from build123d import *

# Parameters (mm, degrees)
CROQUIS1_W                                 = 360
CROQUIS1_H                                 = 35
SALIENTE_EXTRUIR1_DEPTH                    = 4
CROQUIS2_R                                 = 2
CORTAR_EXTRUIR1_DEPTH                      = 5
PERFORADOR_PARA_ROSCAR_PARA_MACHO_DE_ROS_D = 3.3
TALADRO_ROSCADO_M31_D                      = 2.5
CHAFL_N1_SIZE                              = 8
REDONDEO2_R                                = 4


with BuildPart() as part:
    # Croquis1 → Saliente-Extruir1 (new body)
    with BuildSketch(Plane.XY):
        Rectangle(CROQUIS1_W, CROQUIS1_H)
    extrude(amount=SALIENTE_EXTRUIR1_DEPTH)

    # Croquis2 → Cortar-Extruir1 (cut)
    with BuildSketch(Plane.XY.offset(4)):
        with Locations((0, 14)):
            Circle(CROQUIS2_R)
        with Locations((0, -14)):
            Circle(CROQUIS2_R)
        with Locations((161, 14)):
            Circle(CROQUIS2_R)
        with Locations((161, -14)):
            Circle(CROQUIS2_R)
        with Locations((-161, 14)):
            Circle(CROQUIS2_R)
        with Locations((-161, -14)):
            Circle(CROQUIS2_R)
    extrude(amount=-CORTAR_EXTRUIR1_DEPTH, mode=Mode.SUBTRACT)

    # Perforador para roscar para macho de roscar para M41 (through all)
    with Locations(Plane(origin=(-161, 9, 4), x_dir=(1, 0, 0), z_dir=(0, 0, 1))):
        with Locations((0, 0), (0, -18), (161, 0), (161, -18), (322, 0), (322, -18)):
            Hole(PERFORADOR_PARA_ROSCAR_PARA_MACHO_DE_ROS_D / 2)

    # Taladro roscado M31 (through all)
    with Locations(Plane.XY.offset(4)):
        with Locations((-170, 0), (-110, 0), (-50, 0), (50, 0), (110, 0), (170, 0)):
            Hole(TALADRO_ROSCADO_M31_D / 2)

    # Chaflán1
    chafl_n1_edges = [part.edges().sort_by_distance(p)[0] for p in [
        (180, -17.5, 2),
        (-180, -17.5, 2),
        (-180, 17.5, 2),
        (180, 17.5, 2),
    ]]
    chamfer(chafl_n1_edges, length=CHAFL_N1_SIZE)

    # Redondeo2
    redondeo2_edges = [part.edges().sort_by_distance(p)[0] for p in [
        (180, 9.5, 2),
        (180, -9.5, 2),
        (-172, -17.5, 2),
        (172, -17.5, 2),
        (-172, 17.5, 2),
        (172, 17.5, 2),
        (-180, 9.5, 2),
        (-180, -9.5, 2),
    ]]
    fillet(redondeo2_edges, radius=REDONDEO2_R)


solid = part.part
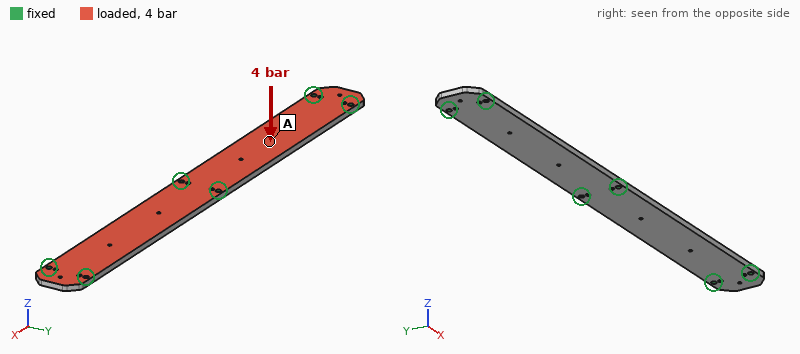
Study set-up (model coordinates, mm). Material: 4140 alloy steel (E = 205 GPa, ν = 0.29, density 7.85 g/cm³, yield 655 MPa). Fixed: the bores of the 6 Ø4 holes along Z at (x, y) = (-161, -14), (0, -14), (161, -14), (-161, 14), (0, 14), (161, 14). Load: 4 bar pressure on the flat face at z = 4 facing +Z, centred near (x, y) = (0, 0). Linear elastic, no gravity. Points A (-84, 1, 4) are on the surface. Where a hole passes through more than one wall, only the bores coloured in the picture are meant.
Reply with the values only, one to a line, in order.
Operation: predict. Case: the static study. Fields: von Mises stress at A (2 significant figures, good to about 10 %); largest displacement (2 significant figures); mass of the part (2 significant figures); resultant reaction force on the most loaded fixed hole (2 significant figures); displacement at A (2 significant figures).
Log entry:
160 MPa
0.65 mm
390 g
1.1 kN
0.64 mm
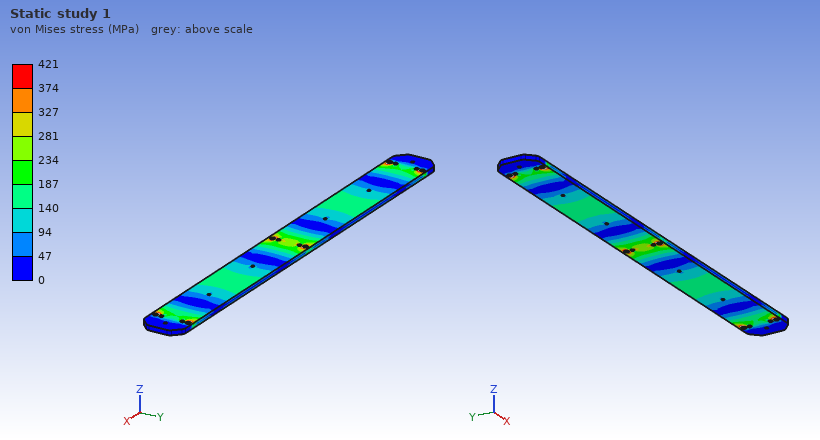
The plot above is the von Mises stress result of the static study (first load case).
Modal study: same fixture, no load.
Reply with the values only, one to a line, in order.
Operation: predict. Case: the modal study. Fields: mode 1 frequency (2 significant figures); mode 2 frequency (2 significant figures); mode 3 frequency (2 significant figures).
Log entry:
780 Hz
810 Hz
2200 Hz
